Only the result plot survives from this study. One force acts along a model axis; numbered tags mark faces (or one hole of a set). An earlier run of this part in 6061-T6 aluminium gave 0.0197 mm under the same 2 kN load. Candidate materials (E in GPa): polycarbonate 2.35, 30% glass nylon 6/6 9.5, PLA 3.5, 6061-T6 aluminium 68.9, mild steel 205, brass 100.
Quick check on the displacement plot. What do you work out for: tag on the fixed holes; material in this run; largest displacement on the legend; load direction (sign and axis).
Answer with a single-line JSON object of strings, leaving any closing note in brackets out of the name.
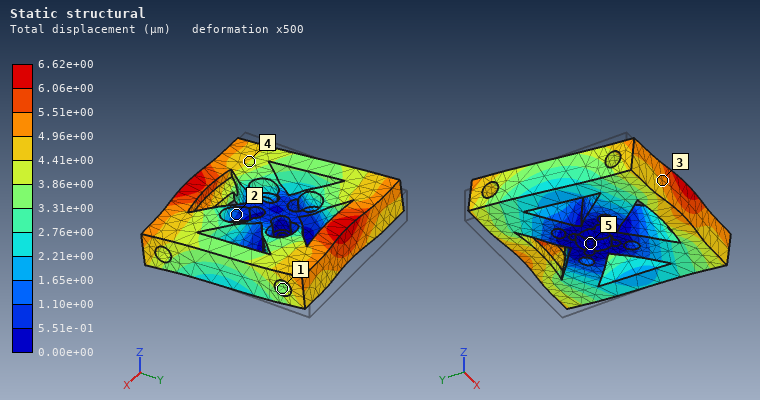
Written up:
{"tag on the fixed holes": "5", "material in this run": "mild steel", "largest displacement on the legend": "6.62e+00 µm", "load direction": "-Y"}
